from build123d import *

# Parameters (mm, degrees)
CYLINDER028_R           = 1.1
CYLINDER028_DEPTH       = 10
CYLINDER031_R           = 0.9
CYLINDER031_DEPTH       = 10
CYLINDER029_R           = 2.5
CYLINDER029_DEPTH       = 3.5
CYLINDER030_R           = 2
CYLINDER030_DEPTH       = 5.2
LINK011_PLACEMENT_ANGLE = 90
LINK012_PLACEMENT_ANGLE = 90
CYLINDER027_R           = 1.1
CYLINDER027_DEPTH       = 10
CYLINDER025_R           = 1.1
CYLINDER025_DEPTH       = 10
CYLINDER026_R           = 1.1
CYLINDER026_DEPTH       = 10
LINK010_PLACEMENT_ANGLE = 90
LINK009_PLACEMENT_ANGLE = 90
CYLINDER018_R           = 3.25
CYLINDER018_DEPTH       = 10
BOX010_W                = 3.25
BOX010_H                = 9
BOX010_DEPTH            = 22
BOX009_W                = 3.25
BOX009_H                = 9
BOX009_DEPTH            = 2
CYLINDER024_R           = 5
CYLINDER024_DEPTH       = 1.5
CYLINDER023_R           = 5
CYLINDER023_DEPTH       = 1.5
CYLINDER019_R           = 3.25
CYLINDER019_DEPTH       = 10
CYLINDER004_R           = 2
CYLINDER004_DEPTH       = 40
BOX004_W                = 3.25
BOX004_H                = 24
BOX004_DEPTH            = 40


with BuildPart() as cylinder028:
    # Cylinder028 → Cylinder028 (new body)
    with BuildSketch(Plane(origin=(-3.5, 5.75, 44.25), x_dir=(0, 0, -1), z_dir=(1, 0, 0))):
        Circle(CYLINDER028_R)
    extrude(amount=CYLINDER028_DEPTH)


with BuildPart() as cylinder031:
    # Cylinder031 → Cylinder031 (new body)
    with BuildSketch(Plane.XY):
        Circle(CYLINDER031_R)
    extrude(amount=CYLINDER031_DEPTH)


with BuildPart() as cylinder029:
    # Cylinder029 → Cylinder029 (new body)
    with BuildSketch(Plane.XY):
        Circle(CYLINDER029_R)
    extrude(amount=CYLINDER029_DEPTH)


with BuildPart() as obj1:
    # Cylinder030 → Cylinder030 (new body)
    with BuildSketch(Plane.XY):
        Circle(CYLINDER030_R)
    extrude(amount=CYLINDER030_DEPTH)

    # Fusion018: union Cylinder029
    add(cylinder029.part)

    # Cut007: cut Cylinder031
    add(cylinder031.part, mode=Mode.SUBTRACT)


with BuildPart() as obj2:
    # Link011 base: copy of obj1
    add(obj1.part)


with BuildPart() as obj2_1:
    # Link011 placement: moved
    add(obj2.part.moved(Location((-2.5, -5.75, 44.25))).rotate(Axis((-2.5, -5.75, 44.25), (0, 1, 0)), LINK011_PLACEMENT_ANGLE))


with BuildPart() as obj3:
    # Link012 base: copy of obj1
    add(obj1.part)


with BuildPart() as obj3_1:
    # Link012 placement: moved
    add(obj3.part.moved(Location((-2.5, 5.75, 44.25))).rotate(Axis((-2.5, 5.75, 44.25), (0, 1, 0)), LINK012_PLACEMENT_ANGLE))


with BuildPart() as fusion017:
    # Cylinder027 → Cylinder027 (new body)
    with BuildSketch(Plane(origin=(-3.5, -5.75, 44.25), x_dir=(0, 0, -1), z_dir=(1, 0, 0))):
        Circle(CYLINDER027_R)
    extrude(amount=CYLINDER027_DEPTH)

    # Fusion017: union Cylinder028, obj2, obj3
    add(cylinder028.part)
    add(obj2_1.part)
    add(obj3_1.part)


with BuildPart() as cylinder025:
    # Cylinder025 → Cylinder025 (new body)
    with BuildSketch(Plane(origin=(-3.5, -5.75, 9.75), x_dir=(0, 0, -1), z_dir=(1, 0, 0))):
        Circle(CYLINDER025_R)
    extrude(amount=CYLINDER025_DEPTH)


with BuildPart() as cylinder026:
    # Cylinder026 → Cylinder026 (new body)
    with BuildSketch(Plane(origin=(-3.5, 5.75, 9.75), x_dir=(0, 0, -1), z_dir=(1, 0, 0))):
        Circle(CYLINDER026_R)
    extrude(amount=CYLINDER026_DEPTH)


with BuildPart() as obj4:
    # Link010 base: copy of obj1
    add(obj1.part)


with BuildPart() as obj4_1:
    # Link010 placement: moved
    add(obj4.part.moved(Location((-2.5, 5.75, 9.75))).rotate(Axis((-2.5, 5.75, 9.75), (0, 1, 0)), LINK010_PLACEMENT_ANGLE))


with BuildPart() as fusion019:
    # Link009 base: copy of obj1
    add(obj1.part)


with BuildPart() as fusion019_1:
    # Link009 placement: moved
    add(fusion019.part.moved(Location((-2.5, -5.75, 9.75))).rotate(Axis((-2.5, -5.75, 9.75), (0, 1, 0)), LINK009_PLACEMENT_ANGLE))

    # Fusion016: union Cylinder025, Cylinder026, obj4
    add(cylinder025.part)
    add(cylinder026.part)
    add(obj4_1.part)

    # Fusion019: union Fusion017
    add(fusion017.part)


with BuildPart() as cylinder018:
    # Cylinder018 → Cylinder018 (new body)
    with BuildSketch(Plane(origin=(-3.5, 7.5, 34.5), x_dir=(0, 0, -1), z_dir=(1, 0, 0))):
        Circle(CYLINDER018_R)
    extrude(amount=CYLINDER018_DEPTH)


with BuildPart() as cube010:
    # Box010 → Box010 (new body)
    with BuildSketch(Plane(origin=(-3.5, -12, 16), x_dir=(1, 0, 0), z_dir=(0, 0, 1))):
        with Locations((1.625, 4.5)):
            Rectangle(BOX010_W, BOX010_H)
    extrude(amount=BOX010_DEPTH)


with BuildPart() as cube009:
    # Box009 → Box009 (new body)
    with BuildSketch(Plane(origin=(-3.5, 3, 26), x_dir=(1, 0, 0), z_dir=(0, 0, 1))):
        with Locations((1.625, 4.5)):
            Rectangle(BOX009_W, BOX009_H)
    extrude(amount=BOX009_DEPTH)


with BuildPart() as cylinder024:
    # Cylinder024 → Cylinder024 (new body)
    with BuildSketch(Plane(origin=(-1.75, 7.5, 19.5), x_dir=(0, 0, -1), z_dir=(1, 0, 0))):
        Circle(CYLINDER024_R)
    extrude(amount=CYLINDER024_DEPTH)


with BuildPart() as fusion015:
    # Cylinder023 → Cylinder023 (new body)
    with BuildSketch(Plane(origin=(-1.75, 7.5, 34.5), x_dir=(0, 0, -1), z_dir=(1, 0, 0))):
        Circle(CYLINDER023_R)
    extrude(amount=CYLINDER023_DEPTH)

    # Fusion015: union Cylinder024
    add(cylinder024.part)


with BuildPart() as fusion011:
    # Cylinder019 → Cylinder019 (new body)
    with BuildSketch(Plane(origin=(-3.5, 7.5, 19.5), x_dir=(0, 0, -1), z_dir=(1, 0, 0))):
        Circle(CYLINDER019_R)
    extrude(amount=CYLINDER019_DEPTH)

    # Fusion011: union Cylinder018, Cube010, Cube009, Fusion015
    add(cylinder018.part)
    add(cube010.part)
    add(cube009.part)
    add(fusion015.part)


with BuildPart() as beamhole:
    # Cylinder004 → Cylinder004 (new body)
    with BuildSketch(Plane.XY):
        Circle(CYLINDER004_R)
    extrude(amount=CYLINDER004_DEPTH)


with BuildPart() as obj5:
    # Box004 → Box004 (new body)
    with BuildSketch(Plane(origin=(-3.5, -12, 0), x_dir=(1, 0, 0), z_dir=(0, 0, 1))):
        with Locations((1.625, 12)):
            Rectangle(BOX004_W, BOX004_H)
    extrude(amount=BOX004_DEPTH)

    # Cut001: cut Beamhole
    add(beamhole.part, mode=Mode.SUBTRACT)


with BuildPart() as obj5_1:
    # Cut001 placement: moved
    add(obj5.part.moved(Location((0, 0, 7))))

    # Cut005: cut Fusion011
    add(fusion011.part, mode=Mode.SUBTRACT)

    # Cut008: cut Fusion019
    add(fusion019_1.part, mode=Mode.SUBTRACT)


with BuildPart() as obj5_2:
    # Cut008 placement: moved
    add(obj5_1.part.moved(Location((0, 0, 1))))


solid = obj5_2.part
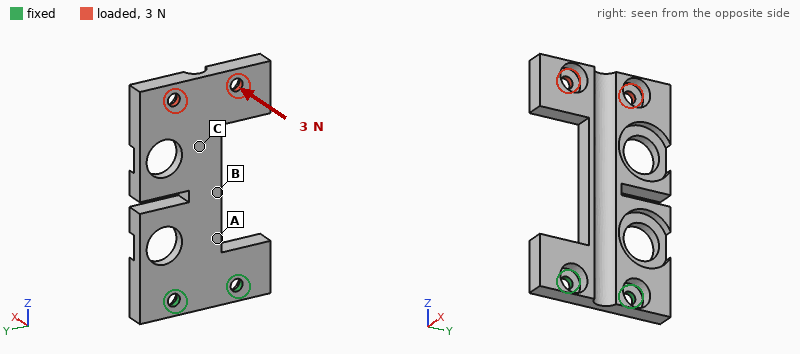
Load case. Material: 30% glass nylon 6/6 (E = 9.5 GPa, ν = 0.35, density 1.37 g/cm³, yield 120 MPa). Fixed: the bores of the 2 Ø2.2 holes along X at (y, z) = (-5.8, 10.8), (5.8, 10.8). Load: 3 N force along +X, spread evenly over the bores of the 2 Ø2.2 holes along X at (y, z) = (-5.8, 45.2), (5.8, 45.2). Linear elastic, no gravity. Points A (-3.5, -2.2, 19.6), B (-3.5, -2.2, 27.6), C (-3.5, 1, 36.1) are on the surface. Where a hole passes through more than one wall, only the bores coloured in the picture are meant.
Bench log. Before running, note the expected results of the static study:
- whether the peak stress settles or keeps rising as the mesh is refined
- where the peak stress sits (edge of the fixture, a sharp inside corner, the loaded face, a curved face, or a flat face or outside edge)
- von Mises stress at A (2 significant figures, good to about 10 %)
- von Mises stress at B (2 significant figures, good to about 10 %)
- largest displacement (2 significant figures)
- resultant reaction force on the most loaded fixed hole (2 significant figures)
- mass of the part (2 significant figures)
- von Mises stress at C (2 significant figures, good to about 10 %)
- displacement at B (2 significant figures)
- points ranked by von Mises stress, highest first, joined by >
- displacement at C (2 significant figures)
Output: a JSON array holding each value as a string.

["keeps rising", "edge of the fixture", "9.1 MPa", "5.9 MPa", "0.45 mm", "3.6 N", "2.3 g", "2.9 MPa", "0.12 mm", "A > B > C", "0.24 mm"]
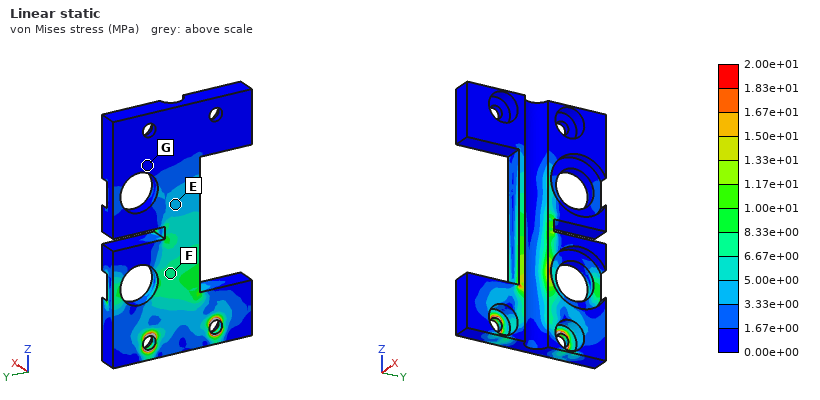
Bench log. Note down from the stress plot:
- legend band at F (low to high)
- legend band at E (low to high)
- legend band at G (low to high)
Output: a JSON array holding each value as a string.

["6.67e+00 to 8.33e+00 MPa", "3.33e+00 to 5.00e+00 MPa", "0.00e+00 to 1.67e+00 MPa"]
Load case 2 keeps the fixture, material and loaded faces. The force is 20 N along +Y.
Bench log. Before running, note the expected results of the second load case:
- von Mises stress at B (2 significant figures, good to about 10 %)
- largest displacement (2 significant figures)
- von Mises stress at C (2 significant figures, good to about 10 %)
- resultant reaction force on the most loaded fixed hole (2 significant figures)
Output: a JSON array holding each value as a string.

["16 MPa", "0.30 mm", "4.2 MPa", "58 N"]
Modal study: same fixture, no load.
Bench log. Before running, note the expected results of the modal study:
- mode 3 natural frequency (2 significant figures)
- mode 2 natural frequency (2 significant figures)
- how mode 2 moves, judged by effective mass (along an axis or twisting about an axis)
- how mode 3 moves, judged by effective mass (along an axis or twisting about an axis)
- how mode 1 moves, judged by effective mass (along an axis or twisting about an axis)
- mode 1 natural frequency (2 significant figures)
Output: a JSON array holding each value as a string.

["1600 Hz", "1300 Hz", "twisting about Z", "along Y", "along X", "510 Hz"]
